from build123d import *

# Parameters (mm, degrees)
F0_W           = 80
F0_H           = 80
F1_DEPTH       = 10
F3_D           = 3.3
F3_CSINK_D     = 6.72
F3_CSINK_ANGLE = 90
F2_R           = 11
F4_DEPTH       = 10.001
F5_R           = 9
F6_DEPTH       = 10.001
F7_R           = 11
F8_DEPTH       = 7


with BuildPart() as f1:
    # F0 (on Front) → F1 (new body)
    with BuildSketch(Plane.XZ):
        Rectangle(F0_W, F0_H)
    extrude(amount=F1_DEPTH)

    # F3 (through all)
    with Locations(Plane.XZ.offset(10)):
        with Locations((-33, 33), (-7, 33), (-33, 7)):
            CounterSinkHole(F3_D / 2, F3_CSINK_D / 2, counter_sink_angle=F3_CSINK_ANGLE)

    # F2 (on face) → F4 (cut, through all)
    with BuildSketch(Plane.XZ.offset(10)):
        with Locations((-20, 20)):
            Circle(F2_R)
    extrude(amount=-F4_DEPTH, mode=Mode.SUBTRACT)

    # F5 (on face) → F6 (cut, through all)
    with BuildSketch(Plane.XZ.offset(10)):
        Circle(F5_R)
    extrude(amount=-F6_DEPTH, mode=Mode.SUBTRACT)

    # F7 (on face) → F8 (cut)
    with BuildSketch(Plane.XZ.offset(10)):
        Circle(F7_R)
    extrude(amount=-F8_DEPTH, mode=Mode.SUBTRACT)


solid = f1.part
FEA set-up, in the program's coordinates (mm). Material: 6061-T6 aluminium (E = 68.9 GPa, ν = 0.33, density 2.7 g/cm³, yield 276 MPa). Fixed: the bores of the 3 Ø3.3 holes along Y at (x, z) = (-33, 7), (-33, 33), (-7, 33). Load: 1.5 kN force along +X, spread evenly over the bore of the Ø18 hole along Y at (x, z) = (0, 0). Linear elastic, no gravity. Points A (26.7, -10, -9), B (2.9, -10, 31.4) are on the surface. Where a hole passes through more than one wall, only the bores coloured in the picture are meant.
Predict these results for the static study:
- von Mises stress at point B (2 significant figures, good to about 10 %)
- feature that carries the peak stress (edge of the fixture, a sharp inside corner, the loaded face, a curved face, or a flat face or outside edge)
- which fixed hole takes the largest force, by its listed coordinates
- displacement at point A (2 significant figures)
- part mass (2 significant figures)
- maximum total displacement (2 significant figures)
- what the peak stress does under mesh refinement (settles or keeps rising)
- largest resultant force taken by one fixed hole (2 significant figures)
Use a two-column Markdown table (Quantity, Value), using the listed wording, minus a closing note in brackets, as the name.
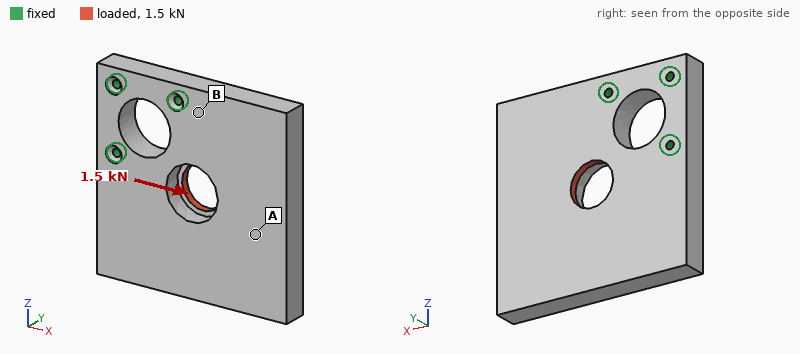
| Quantity | Value |
|---|---|
| von Mises stress at point B | 4.9 MPa |
| feature that carries the peak stress | edge of the fixture |
| which fixed hole takes the largest force, by its listed coordinates | (-33, 7) |
| displacement at point A | 21 µm |
| part mass | 150 g |
| maximum total displacement | 33 µm |
| what the peak stress does under mesh refinement | keeps rising |
| largest resultant force taken by one fixed hole | 1.4 kN |
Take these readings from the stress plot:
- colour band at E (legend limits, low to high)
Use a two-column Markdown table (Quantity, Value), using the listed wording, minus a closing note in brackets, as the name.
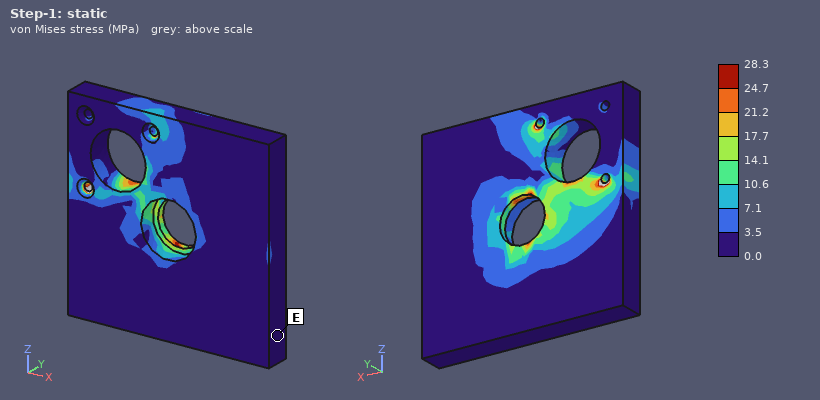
| Quantity | Value |
|---|---|
| colour band at E | 0.0 to 3.5 MPa |
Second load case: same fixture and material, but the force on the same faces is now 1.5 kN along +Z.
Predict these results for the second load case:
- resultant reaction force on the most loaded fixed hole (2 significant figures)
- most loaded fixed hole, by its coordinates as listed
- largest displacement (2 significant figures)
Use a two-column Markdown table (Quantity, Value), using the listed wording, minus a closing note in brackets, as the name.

| Quantity | Value |
|---|---|
| resultant reaction force on the most loaded fixed hole | 1.4 kN |
| most loaded fixed hole, by its coordinates as listed | (-7, 33) |
| largest displacement | 33 µm |
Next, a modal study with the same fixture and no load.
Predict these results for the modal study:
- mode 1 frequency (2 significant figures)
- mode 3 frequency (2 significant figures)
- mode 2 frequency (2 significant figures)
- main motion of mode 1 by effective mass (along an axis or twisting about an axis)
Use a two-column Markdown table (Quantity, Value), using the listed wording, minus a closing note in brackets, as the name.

| Quantity | Value |
|---|---|
| mode 1 frequency | 1200 Hz |
| mode 3 frequency | 3800 Hz |
| mode 2 frequency | 2800 Hz |
| main motion of mode 1 by effective mass | along Y |
